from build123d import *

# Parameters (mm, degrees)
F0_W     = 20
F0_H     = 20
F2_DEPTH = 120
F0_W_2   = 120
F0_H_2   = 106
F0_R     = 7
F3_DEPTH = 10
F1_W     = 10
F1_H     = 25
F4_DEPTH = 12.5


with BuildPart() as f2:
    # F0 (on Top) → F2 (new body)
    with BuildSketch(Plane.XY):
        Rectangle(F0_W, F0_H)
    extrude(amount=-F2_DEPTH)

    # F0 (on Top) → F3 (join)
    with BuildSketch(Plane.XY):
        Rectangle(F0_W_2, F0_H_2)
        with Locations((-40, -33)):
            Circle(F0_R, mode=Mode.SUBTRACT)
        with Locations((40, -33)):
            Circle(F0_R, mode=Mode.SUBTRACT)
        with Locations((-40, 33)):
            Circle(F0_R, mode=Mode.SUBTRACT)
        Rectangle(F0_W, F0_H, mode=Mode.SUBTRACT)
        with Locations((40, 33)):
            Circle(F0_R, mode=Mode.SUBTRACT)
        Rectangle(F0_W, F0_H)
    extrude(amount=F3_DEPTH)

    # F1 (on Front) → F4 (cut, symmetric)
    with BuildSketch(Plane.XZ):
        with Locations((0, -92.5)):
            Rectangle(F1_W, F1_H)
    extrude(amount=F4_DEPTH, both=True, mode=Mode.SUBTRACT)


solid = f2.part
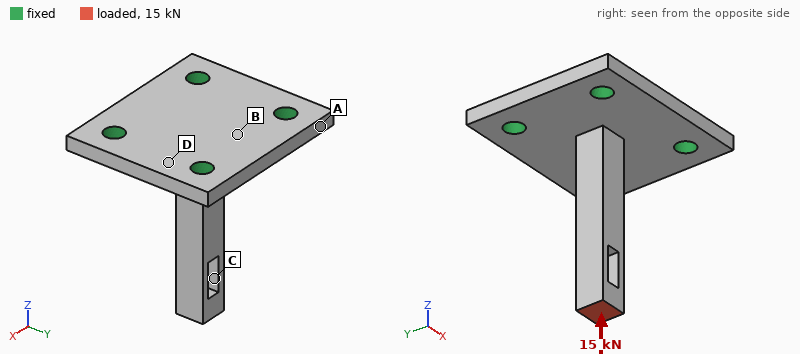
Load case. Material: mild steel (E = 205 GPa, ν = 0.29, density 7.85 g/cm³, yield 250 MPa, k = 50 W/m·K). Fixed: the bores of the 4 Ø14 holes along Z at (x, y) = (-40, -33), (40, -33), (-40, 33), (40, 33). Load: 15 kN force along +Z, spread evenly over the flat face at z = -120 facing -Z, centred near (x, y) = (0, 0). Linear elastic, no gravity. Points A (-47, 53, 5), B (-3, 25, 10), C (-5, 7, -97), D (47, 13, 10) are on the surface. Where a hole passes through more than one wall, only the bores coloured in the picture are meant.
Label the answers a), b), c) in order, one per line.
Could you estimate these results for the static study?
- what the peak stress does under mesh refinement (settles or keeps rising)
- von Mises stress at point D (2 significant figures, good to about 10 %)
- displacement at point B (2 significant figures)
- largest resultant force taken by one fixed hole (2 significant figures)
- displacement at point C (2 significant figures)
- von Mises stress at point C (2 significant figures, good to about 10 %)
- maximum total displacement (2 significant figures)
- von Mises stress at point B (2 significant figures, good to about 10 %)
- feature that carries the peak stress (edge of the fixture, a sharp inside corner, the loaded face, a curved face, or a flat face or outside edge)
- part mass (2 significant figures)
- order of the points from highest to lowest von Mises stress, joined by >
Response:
a) keeps rising
b) 28 MPa
c) 22 µm
d) 3.8 kN
e) 58 µm
f) 88 MPa
g) 65 µm
h) 49 MPa
i) edge of the fixture
j) 1.3 kg
k) C > B > D > A
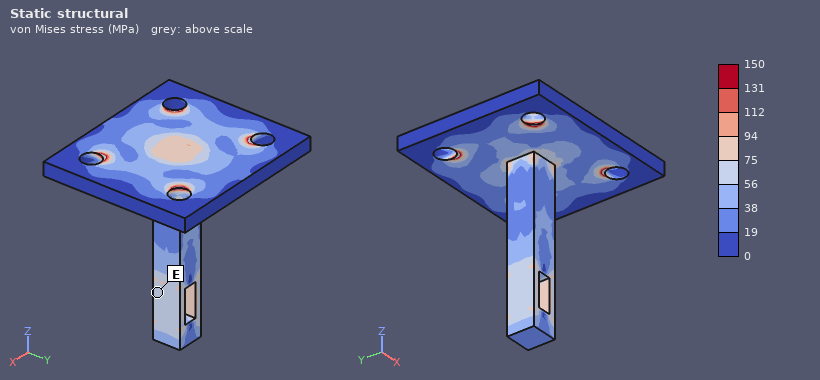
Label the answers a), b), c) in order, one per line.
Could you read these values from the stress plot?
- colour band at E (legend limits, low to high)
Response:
a) 56 to 75 MPa
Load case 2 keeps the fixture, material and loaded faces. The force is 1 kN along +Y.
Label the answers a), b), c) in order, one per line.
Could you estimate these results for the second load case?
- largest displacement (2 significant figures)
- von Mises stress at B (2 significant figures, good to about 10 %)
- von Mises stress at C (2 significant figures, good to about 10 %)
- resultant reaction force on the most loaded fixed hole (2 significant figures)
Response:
a) 0.31 mm
b) 19 MPa
c) 27 MPa
d) 1.2 kN
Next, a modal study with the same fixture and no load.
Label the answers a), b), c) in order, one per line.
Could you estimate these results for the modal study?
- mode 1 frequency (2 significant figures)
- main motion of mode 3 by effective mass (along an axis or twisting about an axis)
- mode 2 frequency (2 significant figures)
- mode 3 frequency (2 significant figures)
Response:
a) 1000 Hz
b) along Z
c) 1000 Hz
d) 4400 Hz
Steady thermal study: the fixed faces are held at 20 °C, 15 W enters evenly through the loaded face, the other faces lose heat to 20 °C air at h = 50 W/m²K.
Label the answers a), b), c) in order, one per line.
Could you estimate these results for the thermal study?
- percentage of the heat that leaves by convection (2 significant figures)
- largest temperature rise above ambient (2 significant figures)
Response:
a) 80 %
b) 57 K
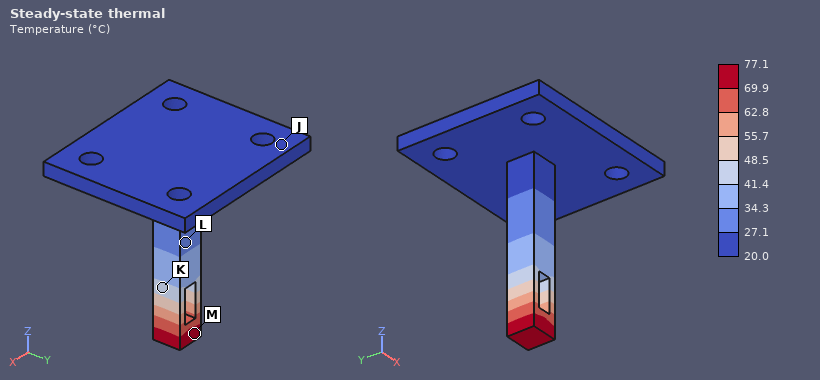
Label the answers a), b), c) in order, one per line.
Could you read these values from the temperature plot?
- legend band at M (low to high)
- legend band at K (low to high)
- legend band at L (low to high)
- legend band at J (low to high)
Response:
a) 69.9 to 77.1 °C
b) 41.4 to 48.5 °C
c) 27.1 to 34.3 °C
d) 20.0 to 27.1 °C
